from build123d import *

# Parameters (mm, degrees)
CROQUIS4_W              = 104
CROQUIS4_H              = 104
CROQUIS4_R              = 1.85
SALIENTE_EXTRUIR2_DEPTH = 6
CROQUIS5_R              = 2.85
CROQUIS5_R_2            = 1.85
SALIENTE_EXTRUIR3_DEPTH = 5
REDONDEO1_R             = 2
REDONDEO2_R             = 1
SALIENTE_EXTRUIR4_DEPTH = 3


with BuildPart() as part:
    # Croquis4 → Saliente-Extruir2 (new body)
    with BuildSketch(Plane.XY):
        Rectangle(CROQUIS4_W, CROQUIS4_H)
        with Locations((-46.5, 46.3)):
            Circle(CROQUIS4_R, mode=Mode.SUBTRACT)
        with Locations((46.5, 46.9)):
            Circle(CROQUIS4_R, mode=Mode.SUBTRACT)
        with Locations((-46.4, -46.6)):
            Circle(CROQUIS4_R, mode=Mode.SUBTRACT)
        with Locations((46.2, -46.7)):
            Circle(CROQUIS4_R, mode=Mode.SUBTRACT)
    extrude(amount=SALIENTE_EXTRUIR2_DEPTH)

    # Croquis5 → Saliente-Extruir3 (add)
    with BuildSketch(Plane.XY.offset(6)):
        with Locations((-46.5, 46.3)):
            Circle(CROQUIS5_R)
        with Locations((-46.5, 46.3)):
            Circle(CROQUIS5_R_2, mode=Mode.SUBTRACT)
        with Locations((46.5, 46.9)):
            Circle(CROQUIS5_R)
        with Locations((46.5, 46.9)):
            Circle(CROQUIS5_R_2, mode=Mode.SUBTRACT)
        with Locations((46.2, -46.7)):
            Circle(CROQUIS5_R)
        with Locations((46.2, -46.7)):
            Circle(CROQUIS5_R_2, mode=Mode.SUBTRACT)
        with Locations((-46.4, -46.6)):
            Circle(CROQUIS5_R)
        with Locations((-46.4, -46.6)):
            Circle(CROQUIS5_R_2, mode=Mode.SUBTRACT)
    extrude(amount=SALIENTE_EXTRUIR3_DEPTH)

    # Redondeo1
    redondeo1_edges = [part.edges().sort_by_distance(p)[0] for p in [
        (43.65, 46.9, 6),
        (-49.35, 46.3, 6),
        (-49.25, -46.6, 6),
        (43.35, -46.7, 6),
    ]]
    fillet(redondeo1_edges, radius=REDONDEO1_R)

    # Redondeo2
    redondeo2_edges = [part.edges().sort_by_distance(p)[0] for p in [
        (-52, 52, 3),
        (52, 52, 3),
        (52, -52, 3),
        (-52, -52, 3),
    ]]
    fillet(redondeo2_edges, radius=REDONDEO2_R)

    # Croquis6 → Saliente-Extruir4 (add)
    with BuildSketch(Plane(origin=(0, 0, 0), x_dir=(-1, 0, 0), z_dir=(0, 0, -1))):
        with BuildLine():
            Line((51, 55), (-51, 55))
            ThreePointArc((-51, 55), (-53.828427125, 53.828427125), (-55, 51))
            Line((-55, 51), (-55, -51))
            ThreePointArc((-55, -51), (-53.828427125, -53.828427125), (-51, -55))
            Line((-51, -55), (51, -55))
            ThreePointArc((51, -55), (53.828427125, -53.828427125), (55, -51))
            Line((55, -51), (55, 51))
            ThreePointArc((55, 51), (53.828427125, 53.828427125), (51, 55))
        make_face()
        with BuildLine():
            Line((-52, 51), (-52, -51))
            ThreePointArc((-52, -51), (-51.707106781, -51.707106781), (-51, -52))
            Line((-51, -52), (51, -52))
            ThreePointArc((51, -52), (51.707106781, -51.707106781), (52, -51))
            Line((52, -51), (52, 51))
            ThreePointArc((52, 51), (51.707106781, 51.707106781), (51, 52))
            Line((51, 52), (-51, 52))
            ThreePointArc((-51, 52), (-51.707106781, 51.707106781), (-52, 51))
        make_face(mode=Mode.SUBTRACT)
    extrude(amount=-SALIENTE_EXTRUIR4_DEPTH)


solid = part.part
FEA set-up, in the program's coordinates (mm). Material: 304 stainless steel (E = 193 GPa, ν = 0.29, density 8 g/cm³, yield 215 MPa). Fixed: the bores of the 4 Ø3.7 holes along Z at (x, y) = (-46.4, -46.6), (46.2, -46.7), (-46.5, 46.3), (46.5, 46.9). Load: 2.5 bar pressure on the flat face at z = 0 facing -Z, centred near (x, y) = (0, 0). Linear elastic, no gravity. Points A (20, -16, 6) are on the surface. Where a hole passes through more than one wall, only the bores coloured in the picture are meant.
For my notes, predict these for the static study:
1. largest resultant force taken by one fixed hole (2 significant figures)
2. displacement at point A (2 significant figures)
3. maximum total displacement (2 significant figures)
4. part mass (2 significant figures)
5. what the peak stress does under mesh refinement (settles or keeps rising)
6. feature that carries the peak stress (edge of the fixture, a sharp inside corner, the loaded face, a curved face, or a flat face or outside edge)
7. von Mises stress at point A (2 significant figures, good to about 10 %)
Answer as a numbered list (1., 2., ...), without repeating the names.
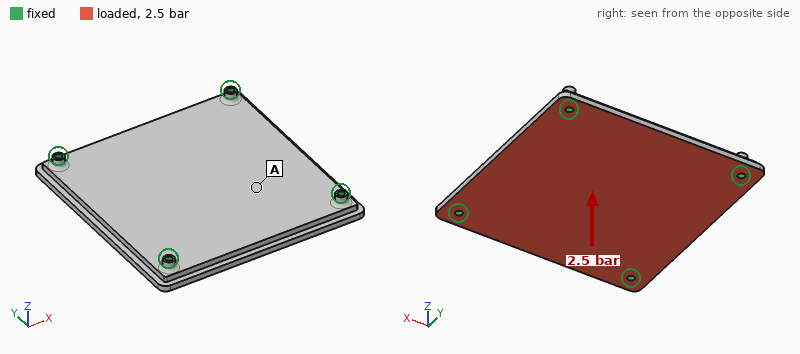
1. 760 N
2. 35 µm
3. 44 µm
4. 550 g
5. keeps rising
6. edge of the fixture
7. 17 MPa
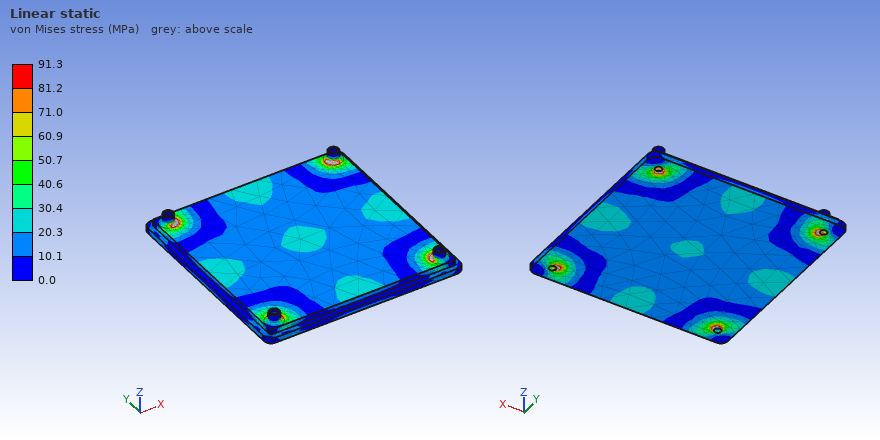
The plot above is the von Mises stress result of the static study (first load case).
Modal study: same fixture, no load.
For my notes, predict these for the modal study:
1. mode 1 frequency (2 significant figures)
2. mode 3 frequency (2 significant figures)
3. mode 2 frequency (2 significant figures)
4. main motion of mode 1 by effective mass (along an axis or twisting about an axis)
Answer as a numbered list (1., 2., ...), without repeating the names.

1. 2100 Hz
2. 3700 Hz
3. 3600 Hz
4. along Z
